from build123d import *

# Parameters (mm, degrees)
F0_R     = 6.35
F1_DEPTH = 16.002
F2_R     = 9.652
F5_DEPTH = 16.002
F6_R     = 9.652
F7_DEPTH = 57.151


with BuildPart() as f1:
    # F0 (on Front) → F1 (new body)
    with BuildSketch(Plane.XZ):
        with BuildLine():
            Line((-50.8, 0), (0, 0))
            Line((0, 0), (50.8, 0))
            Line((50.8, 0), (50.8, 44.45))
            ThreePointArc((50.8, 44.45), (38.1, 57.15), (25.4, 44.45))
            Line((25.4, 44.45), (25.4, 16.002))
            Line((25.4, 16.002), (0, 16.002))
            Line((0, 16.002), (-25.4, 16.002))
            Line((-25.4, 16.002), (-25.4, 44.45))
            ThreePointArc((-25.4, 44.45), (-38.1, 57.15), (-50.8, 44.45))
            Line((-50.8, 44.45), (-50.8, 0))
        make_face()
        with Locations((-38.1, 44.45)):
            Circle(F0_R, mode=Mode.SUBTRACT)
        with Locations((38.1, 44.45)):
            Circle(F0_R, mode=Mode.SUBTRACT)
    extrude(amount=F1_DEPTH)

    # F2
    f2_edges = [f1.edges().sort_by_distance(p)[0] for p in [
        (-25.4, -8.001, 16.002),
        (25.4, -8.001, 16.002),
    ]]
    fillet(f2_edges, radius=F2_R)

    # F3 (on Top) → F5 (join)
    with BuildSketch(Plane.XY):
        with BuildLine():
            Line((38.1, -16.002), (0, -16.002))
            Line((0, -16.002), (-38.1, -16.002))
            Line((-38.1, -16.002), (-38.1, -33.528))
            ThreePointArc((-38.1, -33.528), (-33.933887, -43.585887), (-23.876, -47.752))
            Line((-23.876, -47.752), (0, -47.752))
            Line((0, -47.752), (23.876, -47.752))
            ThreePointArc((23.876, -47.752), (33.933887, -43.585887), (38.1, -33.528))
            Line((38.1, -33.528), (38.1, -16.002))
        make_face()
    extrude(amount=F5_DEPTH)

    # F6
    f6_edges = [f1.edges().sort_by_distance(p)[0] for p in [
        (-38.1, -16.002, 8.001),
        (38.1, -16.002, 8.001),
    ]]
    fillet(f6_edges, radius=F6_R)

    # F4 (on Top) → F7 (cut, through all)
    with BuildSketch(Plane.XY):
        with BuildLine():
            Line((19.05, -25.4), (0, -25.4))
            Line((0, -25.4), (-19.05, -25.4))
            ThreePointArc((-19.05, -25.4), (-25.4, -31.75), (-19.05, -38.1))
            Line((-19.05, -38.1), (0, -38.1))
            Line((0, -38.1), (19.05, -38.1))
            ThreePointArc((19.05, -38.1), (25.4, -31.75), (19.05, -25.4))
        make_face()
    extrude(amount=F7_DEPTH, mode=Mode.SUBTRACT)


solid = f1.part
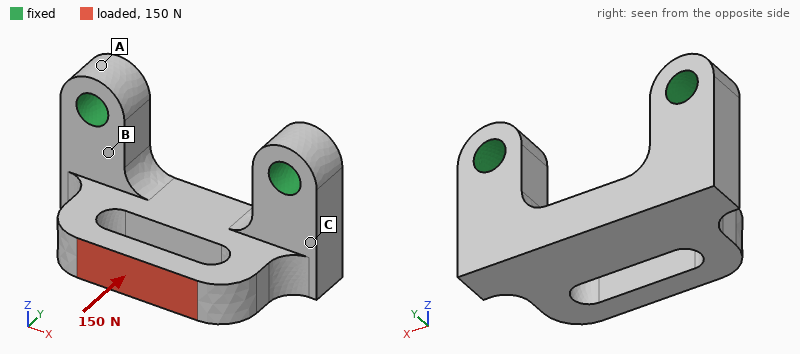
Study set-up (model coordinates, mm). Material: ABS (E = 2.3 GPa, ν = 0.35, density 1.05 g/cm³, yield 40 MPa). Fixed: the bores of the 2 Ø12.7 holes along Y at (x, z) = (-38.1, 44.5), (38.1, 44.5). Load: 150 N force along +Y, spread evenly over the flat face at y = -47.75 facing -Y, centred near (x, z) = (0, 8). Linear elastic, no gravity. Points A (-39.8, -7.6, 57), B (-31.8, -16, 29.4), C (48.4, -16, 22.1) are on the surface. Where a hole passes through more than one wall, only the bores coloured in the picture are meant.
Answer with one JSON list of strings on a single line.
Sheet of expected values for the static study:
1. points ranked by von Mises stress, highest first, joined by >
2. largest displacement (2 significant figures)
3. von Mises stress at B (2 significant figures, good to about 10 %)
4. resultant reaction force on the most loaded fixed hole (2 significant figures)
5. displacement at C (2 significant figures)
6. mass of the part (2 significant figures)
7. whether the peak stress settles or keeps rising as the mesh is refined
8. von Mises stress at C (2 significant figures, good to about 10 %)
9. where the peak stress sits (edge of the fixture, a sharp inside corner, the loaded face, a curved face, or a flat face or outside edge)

["B > C > A", "0.14 mm", "1.5 MPa", "75 N", "0.024 mm", "86 g", "keeps rising", "0.90 MPa", "edge of the fixture"]
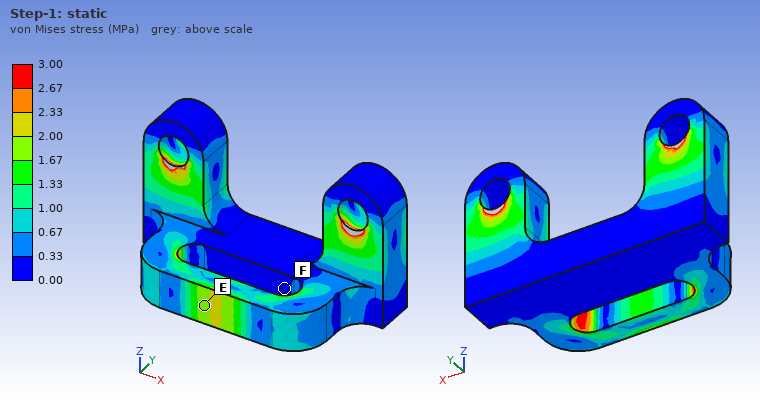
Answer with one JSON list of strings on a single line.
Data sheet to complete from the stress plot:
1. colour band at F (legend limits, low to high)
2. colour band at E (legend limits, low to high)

["0.00 to 0.33 MPa", "1.67 to 2.00 MPa"]
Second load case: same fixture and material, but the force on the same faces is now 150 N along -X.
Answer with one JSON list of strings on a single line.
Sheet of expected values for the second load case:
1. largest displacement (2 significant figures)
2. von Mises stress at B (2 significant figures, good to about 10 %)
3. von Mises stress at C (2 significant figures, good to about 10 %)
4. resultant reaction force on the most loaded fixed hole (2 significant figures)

["82 µm", "0.99 MPa", "0.53 MPa", "110 N"]
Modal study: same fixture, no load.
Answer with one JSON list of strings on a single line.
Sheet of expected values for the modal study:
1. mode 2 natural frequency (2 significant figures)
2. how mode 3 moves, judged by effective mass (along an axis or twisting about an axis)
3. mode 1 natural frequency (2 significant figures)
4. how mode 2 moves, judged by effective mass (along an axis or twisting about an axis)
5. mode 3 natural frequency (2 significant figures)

["1500 Hz", "along Y", "830 Hz", "along X", "1900 Hz"]
